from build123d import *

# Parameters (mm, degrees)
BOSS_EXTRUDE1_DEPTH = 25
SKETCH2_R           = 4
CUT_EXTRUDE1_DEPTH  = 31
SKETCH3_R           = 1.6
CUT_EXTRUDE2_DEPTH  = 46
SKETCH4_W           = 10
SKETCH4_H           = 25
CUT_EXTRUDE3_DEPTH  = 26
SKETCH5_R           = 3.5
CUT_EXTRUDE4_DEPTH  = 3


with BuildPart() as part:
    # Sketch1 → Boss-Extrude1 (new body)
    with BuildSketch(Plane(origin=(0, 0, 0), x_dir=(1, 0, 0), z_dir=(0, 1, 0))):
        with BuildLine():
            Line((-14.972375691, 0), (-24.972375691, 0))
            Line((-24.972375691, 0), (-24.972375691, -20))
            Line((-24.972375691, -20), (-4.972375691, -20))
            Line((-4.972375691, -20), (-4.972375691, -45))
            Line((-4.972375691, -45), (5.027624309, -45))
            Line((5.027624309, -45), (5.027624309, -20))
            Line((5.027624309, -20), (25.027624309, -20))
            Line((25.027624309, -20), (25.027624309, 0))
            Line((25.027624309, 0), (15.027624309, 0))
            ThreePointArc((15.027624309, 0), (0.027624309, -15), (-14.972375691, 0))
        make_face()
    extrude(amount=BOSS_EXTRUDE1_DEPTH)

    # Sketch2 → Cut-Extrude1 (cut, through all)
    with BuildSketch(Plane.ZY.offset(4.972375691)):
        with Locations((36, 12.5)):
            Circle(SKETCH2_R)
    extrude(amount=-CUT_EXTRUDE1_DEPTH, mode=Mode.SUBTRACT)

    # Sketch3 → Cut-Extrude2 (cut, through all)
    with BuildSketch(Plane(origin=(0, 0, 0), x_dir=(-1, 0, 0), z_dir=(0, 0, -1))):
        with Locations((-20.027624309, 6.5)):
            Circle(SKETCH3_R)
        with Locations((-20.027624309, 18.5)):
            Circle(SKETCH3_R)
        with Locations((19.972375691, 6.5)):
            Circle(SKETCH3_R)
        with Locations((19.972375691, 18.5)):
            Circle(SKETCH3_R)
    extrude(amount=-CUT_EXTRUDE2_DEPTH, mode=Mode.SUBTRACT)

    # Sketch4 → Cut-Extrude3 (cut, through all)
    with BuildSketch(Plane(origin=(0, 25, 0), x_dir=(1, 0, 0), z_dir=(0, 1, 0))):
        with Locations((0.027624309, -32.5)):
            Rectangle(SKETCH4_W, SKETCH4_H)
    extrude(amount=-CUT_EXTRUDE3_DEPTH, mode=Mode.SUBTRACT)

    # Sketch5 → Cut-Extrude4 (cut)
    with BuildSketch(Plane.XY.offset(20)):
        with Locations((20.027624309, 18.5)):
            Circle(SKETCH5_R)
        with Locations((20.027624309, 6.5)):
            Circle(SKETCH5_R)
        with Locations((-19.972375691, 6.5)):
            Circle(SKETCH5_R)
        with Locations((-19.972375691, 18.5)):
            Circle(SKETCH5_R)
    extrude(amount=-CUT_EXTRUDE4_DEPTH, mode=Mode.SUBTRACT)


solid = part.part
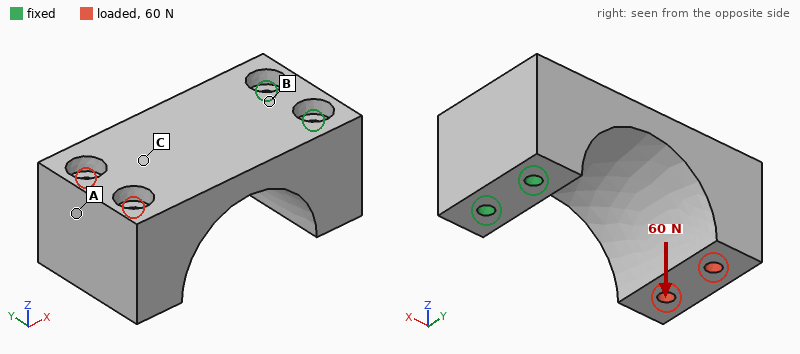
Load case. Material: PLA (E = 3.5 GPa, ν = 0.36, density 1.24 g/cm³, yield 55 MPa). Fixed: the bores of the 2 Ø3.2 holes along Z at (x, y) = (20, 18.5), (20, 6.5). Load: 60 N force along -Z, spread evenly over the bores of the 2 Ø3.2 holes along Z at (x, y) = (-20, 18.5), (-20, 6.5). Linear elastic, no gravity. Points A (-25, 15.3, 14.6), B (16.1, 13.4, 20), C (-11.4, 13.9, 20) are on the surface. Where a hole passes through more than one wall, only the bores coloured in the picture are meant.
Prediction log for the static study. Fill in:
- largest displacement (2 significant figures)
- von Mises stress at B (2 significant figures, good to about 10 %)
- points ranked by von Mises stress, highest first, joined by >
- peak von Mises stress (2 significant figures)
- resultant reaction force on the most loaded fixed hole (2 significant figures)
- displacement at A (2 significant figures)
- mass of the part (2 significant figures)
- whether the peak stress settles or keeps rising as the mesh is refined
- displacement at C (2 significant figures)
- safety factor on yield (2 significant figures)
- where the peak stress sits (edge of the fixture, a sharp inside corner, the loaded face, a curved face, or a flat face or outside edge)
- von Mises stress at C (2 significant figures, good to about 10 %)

0.64 mm
3.6 MPa
B > C > A
12 MPa
31 N
0.55 mm
19 g
settles
0.29 mm
4.7
a flat face or outside edge
2.0 MPa
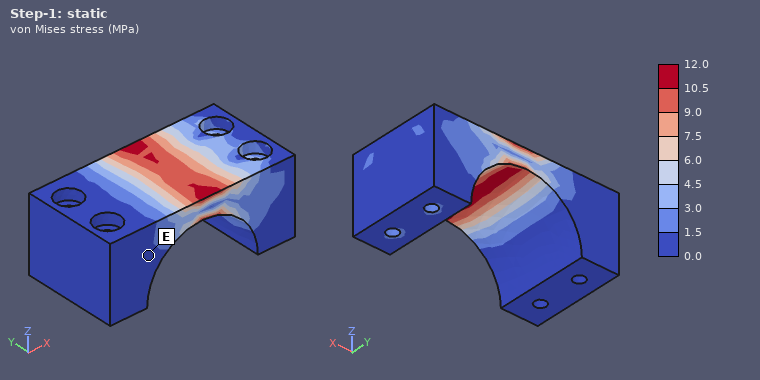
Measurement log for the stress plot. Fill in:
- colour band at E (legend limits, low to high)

0.0 to 1.5 MPa
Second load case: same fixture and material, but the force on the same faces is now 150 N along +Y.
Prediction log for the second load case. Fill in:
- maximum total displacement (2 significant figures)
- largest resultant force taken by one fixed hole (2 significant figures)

0.42 mm
420 N
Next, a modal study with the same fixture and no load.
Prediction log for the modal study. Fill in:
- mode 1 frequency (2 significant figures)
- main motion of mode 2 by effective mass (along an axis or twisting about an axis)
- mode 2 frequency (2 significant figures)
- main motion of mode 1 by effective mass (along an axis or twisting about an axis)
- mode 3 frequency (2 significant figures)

660 Hz
along Y
1400 Hz
along Z
2700 Hz
